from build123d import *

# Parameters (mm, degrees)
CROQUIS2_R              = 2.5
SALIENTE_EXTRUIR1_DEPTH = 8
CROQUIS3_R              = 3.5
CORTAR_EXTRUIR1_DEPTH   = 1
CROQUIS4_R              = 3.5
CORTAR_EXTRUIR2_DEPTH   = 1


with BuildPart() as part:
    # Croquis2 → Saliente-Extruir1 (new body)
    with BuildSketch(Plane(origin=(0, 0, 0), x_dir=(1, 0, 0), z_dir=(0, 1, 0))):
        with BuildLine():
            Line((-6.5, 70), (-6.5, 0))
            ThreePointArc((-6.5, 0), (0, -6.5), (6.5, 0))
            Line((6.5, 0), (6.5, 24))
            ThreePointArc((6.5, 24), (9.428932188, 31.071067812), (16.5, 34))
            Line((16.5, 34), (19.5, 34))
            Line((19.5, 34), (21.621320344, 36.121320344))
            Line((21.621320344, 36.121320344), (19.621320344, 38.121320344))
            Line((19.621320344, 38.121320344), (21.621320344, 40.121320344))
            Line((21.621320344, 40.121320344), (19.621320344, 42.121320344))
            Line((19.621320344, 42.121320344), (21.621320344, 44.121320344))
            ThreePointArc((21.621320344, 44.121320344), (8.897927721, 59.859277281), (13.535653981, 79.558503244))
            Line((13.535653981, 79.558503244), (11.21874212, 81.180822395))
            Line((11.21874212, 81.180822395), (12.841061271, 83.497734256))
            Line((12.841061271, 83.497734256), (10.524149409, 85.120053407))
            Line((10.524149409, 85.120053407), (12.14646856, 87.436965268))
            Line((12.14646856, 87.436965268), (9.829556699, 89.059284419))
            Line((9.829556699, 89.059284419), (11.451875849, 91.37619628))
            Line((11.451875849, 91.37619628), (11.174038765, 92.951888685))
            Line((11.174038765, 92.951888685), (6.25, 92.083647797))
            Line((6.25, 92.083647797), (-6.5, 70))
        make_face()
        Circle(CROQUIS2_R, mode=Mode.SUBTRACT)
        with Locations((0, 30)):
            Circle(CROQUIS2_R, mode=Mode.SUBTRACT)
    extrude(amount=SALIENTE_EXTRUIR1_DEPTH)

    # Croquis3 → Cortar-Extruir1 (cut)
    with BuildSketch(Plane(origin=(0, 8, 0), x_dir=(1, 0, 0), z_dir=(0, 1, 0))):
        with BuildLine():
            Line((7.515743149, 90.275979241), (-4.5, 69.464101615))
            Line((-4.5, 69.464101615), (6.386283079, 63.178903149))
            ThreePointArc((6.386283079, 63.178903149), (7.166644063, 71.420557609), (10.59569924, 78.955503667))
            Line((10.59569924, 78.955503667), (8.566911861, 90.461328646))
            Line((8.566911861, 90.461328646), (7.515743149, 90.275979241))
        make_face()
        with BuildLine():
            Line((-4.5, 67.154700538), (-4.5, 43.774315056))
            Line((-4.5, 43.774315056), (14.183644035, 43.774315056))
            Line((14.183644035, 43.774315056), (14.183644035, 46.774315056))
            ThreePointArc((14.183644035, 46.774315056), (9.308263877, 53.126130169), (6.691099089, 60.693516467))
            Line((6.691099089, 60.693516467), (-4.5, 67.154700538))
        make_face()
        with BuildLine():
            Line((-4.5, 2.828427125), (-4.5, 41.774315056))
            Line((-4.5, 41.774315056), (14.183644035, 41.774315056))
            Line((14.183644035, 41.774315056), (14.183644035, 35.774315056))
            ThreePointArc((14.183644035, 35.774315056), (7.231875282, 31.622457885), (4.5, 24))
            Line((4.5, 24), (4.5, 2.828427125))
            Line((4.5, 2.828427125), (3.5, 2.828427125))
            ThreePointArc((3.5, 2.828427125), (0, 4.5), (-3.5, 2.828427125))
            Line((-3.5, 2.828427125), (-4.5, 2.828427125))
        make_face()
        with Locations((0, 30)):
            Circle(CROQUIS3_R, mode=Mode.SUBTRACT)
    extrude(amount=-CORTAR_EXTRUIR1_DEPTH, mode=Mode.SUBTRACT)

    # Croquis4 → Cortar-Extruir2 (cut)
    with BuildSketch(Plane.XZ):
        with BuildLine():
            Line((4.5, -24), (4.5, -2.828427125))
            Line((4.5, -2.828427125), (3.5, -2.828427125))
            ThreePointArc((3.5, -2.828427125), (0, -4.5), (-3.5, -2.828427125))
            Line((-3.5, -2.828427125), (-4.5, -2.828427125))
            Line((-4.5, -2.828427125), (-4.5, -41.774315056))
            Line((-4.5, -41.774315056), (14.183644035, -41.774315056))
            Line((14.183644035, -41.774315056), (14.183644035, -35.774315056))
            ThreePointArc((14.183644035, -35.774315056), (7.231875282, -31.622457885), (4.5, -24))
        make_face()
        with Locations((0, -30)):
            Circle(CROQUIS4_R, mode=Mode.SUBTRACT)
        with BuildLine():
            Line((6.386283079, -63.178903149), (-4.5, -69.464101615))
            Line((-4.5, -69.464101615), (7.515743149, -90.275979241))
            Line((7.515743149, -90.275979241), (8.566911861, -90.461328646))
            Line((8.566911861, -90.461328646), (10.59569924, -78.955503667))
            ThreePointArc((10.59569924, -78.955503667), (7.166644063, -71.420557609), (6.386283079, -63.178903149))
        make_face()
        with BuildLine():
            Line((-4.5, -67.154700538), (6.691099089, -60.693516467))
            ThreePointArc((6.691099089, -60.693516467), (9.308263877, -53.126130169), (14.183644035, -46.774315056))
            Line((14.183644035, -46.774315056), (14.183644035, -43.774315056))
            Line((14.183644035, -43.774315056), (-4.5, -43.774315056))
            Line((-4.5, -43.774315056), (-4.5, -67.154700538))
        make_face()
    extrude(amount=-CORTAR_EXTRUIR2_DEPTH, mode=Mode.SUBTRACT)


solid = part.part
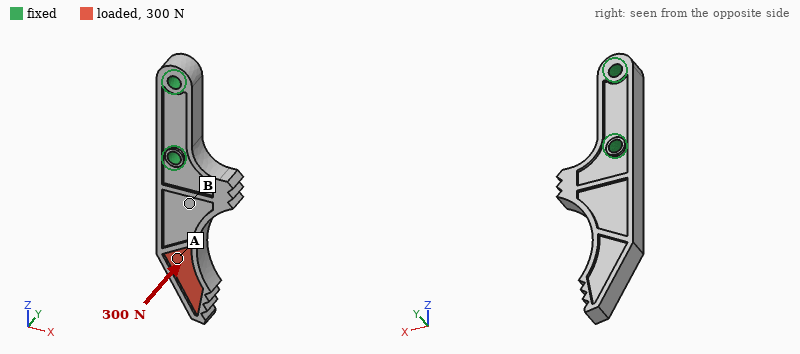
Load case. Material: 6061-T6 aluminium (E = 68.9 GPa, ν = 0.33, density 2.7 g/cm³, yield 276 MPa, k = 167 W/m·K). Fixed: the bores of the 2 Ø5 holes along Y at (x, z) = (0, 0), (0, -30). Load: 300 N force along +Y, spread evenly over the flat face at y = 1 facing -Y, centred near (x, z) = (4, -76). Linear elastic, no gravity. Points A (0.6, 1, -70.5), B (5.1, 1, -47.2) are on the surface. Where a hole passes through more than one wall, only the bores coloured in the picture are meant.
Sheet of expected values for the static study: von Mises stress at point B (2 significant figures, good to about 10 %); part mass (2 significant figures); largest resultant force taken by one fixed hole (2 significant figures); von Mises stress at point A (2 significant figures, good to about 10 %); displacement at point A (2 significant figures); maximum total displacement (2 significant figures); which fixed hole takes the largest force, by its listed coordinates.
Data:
57 MPa
27 g
350 N
18 MPa
0.28 mm
0.54 mm
(0, -30)
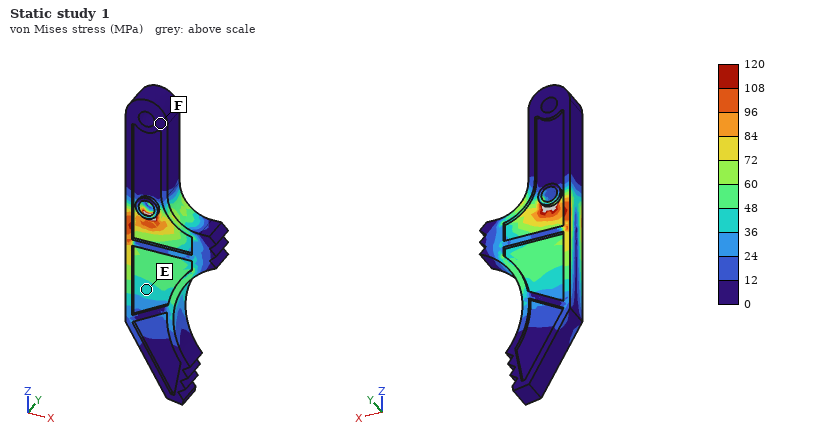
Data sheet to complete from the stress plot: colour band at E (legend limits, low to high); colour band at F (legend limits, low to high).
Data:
36 to 48 MPa
0 to 12 MPa
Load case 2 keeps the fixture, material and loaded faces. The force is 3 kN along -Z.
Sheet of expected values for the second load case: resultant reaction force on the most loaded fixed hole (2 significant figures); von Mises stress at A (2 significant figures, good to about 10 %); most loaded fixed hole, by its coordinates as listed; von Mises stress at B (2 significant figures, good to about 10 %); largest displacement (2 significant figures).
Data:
2.8 kN
86 MPa
(0, -30)
91 MPa
0.61 mm
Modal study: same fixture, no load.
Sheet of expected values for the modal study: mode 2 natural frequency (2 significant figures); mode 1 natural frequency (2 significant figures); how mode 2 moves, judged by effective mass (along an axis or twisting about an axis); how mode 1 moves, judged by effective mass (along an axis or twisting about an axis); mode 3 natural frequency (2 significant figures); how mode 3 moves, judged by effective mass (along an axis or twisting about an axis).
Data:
3400 Hz
1700 Hz
along X
along Y
7700 Hz
twisting about Z
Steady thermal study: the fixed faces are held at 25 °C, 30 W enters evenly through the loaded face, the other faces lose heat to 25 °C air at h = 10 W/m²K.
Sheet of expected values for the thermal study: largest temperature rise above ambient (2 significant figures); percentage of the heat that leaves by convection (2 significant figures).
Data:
76 K
4.5 %
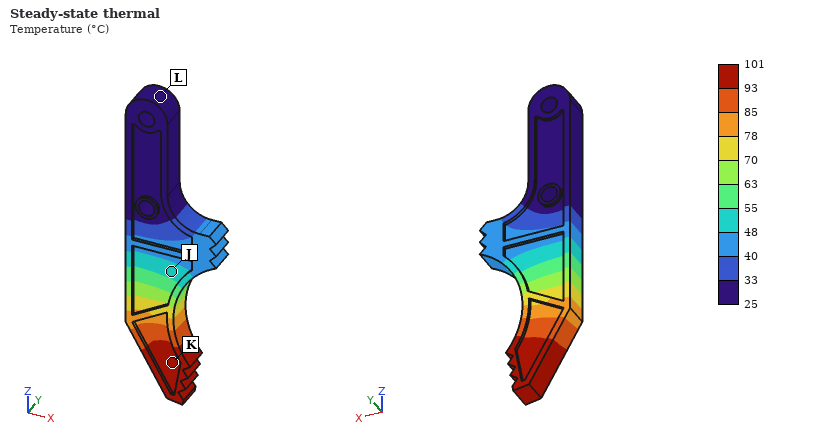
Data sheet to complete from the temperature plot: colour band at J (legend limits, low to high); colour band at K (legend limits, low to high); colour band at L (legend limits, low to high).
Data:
48 to 55 °C
93 to 101 °C
25 to 33 °C
